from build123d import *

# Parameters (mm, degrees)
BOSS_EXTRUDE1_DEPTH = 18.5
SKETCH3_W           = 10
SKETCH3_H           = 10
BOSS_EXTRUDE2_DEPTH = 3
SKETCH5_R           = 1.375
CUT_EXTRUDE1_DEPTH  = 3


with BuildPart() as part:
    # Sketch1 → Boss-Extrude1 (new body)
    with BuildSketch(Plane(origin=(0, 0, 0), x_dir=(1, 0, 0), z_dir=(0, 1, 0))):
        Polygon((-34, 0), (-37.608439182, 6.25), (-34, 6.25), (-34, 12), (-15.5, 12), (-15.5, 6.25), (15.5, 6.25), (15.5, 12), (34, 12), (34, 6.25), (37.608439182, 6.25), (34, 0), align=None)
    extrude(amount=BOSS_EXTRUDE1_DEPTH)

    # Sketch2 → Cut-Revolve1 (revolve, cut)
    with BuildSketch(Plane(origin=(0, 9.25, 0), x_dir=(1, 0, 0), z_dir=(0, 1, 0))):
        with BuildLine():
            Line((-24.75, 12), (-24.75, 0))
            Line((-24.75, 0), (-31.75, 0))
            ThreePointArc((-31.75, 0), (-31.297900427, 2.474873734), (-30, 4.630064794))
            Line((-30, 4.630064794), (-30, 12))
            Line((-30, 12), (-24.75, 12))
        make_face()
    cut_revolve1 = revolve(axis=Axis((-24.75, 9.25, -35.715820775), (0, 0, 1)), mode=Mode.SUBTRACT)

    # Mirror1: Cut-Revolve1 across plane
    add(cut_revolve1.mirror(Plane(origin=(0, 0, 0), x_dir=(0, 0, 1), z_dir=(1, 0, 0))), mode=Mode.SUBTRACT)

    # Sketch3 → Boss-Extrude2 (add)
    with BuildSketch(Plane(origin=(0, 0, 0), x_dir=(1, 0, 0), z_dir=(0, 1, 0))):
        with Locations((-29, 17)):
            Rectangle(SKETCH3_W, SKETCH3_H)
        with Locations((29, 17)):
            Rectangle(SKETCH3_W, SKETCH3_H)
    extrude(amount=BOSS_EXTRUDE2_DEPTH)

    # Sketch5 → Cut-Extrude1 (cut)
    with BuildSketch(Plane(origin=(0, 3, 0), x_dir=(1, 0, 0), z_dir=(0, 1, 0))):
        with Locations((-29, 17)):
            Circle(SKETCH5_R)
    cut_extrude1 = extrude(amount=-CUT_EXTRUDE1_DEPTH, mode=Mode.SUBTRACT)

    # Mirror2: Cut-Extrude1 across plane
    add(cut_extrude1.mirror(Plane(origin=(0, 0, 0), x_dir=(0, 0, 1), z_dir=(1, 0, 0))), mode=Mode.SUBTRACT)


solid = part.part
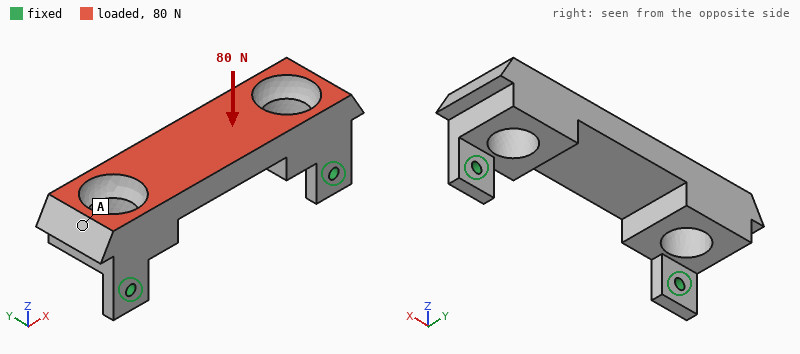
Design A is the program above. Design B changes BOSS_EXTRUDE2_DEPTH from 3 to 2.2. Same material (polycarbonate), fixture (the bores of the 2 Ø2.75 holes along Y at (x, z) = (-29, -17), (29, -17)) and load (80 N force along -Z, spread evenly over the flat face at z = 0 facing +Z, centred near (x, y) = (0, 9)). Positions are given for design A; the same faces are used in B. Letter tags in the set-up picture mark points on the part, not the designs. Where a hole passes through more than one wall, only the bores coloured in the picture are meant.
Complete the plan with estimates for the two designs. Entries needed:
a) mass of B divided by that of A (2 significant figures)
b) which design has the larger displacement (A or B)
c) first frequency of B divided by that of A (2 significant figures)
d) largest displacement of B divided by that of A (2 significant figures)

0.99
B
0.66
2.3
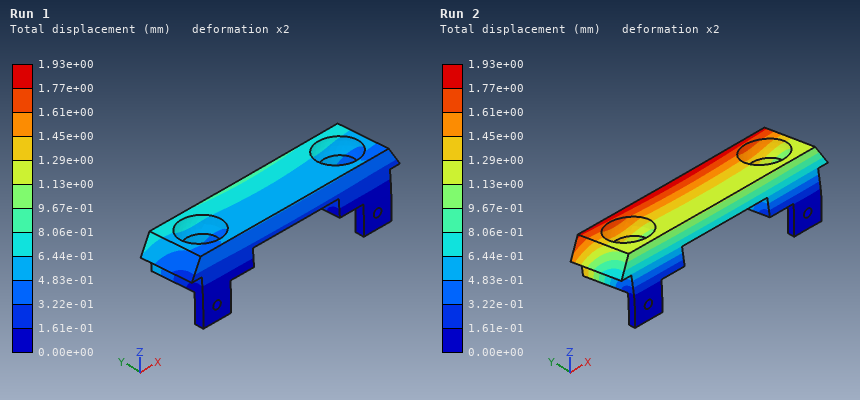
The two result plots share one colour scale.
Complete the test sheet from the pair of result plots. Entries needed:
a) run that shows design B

Run 2
